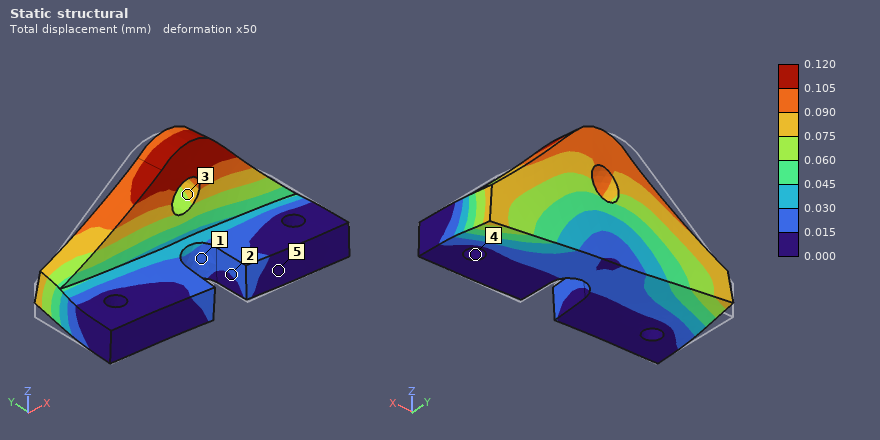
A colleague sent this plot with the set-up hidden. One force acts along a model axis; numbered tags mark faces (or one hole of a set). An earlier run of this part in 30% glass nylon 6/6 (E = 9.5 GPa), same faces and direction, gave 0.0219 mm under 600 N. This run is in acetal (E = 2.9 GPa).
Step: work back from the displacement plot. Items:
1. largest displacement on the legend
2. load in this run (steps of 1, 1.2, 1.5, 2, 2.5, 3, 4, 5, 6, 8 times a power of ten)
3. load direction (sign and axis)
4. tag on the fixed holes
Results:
0.120 mm
1 kN
+X
4
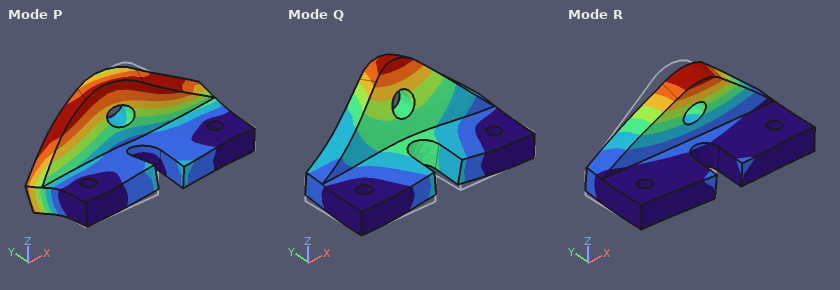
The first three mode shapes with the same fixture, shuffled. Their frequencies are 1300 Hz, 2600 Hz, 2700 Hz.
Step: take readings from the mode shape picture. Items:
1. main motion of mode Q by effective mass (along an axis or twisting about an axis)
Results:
along Z
